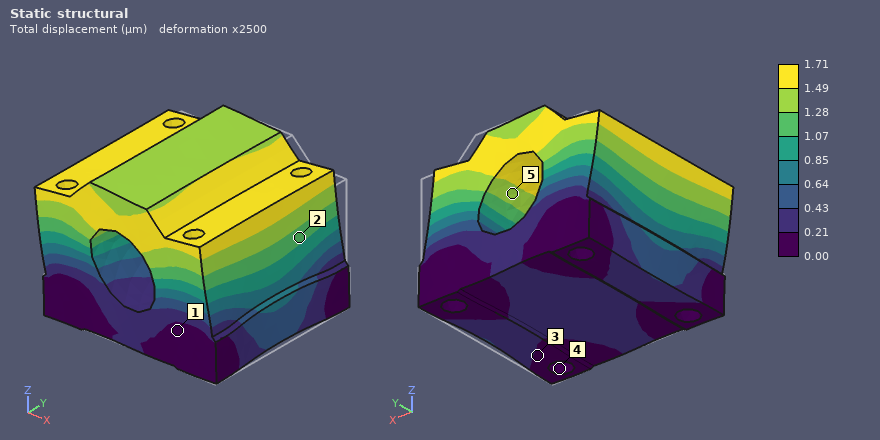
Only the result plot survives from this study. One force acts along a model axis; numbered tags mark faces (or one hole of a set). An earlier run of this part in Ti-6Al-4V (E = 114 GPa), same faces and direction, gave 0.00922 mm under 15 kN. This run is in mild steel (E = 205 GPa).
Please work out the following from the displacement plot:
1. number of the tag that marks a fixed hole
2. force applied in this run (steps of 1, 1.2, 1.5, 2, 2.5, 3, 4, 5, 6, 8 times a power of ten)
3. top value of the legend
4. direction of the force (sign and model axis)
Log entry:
4
5 kN
1.71 µm
-X
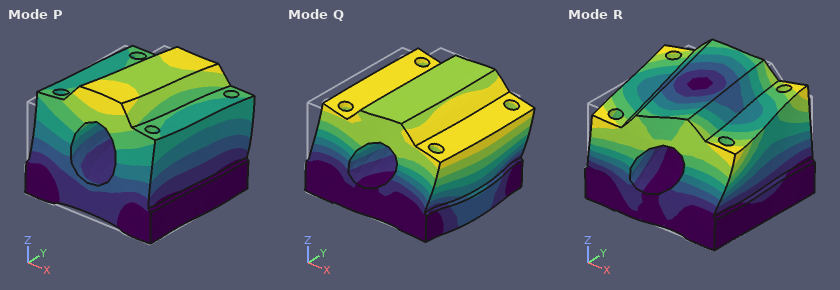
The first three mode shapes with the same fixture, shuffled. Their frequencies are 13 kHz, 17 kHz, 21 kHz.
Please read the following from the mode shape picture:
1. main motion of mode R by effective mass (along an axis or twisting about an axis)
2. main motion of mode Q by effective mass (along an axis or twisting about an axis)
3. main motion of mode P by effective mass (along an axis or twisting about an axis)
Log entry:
twisting about Z
along X
along Y
